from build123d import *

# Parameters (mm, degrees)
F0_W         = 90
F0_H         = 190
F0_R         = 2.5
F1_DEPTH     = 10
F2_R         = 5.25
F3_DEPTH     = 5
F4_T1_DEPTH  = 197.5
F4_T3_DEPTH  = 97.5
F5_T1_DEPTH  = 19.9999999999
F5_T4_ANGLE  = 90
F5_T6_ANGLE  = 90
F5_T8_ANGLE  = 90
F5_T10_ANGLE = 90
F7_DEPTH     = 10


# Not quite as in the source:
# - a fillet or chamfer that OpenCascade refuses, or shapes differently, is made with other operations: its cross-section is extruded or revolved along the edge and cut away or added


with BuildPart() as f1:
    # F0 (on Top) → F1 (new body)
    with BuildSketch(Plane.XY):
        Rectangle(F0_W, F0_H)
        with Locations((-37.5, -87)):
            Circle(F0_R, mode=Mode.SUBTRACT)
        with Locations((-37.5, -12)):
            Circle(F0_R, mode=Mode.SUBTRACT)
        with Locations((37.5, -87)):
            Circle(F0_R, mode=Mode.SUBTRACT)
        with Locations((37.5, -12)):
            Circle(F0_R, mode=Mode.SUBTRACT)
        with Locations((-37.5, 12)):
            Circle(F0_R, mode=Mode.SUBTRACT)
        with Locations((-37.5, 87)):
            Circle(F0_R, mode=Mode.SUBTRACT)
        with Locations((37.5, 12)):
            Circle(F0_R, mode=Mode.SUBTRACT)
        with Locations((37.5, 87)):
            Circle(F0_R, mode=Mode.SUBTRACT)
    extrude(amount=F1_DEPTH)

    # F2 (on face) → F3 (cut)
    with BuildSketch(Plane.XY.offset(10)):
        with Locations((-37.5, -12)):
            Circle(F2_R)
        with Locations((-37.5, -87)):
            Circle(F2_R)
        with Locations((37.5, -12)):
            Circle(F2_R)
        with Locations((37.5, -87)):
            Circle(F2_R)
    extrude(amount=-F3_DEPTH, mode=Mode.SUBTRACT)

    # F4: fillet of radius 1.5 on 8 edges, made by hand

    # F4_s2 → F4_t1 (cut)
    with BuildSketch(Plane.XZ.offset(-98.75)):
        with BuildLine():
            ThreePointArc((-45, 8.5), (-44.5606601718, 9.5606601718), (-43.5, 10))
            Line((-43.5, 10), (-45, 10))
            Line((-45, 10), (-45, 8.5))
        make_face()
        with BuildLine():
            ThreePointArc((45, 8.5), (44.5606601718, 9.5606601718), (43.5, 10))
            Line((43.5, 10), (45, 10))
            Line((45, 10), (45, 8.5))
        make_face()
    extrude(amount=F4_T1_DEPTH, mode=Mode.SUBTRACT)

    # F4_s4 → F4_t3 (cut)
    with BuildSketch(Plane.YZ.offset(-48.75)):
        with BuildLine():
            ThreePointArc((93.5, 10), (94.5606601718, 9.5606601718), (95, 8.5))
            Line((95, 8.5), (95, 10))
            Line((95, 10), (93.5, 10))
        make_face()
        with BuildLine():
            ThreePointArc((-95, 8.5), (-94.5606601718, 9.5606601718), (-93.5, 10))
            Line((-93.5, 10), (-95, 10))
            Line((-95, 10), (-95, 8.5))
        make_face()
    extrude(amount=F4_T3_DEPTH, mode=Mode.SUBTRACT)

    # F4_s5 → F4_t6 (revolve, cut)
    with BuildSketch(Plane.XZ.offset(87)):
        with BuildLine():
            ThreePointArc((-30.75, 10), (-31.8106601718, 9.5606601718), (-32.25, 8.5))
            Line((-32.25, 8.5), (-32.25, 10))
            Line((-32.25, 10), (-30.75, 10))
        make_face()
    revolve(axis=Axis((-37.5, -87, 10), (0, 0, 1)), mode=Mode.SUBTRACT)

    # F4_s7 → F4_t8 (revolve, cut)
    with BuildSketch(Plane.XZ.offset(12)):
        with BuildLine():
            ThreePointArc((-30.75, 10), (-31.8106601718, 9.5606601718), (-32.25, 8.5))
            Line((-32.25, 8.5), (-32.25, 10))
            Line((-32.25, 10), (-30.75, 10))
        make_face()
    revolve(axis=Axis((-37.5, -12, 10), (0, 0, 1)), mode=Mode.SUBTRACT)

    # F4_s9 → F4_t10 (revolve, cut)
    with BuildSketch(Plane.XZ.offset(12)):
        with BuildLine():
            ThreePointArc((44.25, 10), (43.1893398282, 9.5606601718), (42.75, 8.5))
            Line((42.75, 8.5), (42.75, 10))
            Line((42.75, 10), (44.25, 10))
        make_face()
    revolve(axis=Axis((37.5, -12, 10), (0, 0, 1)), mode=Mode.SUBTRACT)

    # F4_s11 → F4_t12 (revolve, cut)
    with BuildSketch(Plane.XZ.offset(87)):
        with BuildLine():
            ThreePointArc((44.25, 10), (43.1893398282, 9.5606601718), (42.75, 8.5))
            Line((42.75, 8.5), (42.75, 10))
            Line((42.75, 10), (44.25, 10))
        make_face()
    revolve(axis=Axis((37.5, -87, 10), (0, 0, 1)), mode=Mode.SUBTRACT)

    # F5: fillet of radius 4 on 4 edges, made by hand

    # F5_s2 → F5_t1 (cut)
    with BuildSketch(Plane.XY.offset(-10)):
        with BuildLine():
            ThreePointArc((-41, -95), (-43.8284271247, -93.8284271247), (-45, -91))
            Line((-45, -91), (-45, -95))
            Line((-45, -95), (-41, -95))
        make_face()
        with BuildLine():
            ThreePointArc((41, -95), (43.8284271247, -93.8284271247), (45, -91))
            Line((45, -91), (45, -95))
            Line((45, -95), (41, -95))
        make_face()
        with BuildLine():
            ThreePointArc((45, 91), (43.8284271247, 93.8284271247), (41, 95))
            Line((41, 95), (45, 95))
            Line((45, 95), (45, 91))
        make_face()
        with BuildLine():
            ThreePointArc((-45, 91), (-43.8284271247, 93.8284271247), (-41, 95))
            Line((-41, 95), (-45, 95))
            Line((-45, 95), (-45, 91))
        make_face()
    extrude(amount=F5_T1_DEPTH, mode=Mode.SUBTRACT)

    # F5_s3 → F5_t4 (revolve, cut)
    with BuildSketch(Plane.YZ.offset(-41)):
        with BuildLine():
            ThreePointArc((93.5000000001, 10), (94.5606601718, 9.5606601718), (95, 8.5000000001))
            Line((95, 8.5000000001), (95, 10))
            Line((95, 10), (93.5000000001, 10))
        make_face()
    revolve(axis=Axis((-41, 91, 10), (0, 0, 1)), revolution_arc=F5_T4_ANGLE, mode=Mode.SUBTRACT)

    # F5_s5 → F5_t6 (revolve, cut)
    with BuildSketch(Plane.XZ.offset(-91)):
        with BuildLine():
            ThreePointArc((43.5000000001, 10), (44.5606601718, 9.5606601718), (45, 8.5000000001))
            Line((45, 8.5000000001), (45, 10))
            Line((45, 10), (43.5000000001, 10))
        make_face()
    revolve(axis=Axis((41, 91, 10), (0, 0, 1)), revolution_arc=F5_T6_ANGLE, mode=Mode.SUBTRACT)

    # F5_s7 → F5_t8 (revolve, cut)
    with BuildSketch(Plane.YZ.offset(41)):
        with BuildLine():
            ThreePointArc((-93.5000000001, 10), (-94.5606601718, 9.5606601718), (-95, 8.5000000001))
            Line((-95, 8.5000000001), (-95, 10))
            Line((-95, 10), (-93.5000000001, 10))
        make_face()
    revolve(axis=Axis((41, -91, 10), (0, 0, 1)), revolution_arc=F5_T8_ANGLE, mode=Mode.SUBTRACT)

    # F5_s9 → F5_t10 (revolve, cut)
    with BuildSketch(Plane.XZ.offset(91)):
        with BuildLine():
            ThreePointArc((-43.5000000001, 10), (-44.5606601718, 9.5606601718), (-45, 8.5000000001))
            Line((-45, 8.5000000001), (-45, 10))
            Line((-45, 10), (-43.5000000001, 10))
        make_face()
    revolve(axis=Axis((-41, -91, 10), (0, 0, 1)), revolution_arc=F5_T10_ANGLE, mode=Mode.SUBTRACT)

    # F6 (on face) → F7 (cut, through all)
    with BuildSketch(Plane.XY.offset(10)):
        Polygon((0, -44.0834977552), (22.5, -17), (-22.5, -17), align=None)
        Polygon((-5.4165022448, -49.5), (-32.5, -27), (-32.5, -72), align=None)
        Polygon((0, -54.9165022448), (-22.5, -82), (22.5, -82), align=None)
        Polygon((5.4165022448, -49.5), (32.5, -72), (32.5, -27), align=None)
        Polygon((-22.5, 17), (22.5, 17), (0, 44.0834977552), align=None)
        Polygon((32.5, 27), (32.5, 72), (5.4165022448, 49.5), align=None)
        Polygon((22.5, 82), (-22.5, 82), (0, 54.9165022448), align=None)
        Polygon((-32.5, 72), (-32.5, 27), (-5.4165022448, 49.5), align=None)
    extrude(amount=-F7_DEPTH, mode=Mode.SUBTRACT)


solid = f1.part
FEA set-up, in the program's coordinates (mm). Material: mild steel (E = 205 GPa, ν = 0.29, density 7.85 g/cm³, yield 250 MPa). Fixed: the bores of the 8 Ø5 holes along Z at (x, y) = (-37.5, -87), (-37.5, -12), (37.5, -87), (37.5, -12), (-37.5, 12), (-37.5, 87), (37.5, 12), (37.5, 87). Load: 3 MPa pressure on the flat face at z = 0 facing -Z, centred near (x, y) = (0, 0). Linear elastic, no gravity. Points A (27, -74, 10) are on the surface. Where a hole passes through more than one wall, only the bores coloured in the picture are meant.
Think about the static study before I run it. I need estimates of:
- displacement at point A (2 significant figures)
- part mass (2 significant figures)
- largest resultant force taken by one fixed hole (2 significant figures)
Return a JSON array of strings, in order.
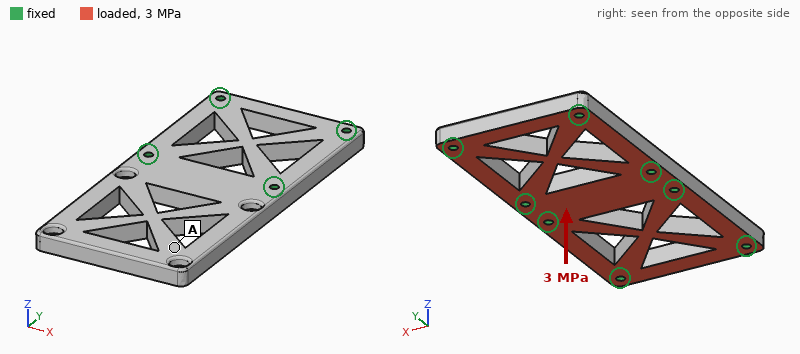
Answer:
["30 µm", "930 g", "6.0 kN"]
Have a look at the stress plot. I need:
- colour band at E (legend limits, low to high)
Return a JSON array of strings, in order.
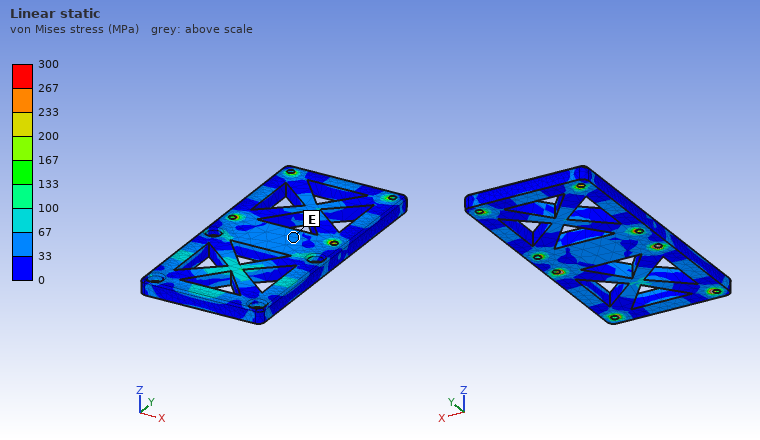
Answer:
["33 to 67 MPa"]
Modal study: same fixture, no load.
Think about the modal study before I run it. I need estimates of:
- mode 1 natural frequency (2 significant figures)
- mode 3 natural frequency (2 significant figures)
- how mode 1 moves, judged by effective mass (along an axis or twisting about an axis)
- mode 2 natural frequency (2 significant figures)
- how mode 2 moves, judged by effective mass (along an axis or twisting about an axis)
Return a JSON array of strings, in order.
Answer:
["4800 Hz", "7300 Hz", "along Z", "5800 Hz", "along Z"]
